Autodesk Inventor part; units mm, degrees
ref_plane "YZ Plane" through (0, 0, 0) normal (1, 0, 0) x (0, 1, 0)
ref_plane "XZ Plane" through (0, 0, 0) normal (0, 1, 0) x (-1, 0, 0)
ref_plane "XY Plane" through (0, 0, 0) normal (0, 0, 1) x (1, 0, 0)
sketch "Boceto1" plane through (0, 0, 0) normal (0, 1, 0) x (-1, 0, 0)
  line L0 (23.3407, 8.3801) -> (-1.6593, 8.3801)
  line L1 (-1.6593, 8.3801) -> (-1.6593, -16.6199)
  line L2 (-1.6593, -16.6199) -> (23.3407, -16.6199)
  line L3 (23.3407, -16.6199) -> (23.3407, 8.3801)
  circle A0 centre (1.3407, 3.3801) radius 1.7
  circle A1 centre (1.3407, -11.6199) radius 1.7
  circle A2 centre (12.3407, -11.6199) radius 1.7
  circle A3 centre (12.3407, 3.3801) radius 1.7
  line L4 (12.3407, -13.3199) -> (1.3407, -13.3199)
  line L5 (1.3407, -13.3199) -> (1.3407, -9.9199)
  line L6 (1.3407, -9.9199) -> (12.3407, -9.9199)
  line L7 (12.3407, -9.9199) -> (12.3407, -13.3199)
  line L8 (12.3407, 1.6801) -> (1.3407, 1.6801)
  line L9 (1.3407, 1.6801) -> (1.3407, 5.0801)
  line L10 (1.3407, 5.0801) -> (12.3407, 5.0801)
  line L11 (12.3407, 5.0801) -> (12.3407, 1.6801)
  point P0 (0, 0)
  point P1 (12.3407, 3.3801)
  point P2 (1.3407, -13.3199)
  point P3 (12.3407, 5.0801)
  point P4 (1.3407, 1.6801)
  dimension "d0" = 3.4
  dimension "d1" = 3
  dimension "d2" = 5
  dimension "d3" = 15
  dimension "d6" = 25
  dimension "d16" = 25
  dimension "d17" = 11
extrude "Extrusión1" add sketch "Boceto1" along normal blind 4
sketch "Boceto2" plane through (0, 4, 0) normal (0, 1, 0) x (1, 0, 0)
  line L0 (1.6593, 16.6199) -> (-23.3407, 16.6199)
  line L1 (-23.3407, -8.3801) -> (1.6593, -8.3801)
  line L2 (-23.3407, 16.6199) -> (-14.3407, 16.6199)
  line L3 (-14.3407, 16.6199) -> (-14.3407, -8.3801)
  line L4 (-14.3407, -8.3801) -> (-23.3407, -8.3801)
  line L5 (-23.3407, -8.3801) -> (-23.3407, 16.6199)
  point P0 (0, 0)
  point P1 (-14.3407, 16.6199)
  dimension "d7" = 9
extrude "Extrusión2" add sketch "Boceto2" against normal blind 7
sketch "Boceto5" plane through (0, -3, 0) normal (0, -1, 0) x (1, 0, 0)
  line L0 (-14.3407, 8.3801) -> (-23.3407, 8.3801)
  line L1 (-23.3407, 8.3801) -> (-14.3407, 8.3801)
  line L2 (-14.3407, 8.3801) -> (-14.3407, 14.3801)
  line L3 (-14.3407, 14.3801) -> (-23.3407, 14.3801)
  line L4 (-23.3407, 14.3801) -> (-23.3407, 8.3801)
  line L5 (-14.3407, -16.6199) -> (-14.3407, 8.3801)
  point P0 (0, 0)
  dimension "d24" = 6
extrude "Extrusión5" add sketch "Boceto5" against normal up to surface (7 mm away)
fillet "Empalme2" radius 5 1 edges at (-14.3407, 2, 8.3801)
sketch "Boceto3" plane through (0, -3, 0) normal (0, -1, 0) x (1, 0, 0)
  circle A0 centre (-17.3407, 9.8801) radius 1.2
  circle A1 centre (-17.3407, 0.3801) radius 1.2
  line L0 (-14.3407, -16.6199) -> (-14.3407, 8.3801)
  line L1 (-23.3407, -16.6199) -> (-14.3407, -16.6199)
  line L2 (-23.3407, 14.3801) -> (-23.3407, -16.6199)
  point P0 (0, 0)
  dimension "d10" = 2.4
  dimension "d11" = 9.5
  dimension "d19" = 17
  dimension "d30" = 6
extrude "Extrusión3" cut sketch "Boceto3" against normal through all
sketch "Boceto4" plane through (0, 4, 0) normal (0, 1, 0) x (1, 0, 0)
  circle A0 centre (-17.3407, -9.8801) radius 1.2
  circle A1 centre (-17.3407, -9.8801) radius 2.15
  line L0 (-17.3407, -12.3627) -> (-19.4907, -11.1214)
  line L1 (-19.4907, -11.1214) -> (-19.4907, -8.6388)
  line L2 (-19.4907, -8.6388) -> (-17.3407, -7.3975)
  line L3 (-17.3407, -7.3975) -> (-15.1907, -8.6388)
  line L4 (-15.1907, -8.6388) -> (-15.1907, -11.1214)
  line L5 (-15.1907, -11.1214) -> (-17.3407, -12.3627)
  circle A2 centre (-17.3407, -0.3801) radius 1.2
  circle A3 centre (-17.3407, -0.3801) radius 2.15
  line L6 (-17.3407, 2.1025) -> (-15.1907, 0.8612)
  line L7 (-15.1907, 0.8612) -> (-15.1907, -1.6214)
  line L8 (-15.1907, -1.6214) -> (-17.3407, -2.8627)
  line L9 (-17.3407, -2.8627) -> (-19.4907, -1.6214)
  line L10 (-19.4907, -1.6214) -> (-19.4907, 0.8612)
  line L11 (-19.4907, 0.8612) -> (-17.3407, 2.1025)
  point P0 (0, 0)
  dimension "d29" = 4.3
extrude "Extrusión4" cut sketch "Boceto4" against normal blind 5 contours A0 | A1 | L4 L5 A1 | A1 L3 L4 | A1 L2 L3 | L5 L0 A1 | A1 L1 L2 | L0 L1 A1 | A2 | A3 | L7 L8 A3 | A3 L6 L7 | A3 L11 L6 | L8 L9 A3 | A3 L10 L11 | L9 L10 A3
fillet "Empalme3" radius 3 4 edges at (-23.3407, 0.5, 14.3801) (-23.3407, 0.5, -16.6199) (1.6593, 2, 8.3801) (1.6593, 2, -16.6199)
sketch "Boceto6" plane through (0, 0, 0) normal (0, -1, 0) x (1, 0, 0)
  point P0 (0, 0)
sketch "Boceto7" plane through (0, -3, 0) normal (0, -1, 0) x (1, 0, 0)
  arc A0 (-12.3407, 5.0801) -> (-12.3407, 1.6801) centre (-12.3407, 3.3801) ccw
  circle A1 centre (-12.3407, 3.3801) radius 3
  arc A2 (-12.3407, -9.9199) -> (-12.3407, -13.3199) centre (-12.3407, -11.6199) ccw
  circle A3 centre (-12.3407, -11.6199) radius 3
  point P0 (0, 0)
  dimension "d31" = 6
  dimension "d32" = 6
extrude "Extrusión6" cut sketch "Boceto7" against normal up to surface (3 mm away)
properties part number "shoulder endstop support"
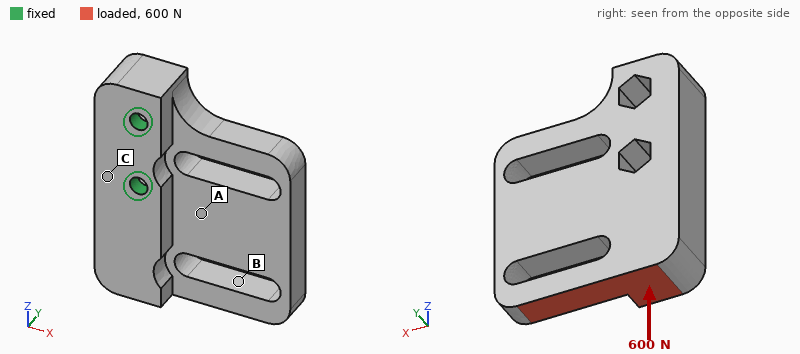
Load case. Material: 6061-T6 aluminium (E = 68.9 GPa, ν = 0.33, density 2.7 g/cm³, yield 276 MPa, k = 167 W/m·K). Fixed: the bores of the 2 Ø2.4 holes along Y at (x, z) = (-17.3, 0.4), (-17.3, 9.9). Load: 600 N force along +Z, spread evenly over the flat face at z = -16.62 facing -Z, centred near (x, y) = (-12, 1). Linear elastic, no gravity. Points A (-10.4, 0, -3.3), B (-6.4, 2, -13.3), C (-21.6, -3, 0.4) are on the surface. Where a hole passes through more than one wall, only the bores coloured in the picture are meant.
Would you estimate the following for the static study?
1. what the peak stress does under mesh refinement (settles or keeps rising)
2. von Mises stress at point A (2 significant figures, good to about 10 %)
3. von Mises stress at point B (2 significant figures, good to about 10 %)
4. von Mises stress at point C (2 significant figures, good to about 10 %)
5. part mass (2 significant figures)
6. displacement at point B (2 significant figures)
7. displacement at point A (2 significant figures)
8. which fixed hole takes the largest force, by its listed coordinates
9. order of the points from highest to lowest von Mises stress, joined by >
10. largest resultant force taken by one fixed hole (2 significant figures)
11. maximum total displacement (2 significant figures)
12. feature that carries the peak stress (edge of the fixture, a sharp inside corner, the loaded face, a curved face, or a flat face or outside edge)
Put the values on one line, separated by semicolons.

keeps rising; 8.6 MPa; 48 MPa; 24 MPa; 8.0 g; 35 µm; 11 µm; (-17.3, 0.4); B > C > A; 520 N; 39 µm; edge of the fixture
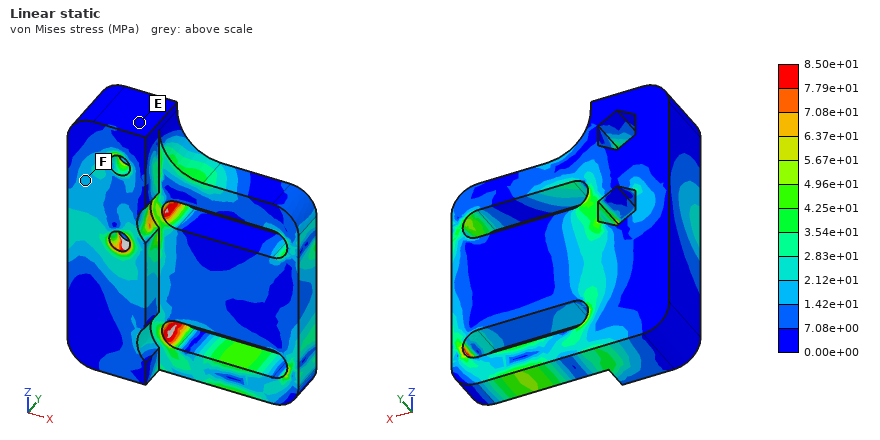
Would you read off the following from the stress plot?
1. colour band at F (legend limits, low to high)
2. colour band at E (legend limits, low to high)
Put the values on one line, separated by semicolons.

1.42e+01 to 2.12e+01 MPa; 0.00e+00 to 7.08e+00 MPa
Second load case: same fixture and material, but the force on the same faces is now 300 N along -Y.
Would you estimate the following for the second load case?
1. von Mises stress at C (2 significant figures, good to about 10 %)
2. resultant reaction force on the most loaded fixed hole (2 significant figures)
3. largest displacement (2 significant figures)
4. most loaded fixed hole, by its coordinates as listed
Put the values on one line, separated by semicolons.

45 MPa; 800 N; 0.12 mm; (-17.3, 0.4)
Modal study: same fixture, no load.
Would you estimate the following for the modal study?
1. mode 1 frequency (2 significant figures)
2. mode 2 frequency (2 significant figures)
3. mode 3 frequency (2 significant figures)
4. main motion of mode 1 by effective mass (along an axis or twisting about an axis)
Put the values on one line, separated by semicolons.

5300 Hz; 8400 Hz; 10 kHz; along Y
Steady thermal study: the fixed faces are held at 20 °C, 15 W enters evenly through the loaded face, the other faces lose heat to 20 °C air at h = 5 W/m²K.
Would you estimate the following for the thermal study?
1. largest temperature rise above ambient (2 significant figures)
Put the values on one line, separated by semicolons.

38 K
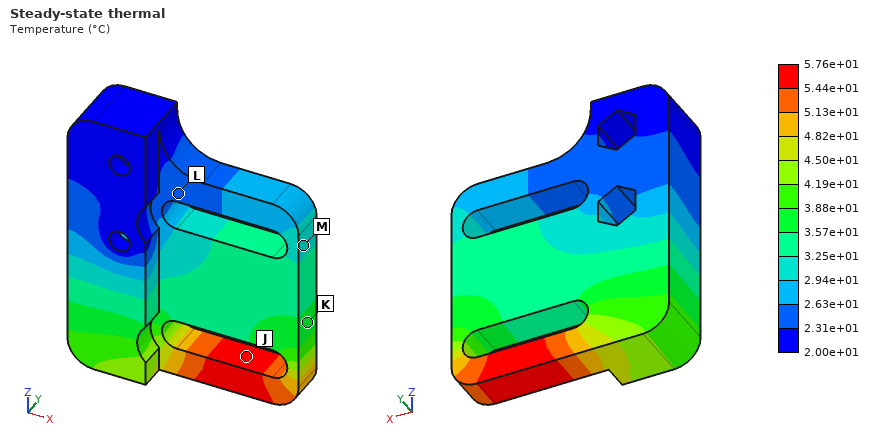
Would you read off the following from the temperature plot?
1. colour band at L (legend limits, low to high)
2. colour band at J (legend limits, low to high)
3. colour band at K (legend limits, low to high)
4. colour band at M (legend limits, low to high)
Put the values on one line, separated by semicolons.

2.31e+01 to 2.63e+01 °C; 5.44e+01 to 5.76e+01 °C; 3.57e+01 to 3.88e+01 °C; 2.94e+01 to 3.25e+01 °C
